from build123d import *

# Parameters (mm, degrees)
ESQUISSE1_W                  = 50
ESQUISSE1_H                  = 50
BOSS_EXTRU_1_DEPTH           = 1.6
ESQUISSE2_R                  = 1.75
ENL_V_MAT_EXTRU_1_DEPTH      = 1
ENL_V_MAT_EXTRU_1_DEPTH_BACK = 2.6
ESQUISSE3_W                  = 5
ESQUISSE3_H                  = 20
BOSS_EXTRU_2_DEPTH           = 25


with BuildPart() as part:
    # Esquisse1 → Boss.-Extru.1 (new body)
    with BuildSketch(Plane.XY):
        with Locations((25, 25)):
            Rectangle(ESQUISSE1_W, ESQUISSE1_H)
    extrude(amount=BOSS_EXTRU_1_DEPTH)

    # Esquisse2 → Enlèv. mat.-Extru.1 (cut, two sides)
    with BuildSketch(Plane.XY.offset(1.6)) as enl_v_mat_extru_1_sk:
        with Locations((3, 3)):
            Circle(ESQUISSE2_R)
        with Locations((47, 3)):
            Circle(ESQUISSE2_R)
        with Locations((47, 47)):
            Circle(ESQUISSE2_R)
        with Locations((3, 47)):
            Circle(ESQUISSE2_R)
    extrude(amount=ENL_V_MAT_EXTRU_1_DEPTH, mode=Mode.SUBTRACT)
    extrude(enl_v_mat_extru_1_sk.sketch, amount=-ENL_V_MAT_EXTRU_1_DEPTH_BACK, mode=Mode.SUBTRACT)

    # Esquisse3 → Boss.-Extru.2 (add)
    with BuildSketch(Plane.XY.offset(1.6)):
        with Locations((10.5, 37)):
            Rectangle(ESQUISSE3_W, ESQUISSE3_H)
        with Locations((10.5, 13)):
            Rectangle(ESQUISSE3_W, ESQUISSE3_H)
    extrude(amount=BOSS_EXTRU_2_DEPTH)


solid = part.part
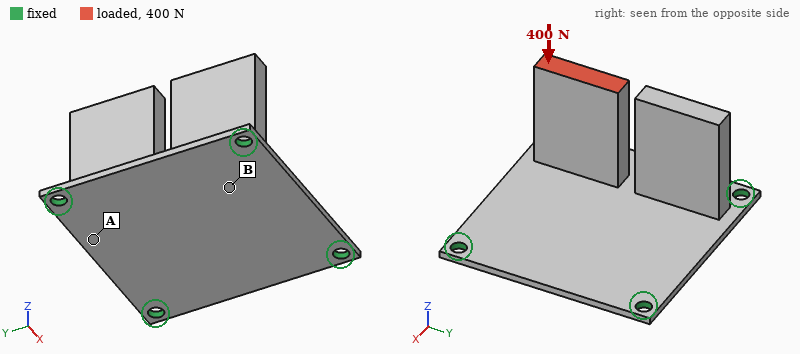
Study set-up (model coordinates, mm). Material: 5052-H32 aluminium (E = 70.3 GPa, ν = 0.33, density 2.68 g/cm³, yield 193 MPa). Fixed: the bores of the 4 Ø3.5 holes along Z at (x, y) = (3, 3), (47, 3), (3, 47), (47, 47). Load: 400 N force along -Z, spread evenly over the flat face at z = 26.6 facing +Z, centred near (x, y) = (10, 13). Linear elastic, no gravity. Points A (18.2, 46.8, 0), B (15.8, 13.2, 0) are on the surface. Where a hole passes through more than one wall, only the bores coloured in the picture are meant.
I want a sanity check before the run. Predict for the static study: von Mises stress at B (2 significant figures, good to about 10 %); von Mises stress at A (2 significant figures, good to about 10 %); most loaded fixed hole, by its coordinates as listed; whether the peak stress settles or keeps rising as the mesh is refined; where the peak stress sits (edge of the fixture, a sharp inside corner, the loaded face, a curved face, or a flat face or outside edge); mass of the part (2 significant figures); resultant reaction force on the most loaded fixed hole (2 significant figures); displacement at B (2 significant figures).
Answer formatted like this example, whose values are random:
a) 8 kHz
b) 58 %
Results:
a) 47 MPa
b) 20 MPa
c) (3, 3)
d) keeps rising
e) edge of the fixture
f) 24 g
g) 290 N
h) 0.12 mm
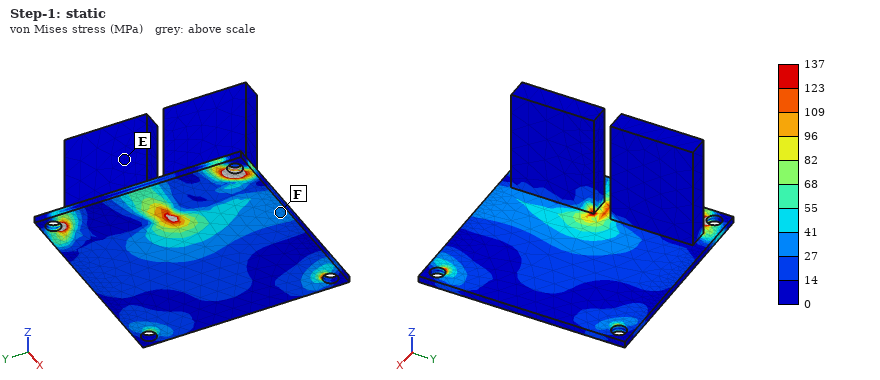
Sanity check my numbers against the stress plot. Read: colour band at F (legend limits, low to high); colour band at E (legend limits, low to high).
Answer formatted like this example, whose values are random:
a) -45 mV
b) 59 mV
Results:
a) 27 to 41 MPa
b) 0 to 14 MPa
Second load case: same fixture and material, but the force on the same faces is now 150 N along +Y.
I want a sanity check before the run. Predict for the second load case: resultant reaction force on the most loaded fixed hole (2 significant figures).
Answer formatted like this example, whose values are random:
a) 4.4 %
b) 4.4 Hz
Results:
a) 120 N
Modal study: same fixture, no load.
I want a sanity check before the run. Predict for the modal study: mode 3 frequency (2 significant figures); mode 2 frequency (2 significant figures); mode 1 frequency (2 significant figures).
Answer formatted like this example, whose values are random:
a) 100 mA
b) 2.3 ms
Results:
a) 2300 Hz
b) 1800 Hz
c) 1400 Hz
